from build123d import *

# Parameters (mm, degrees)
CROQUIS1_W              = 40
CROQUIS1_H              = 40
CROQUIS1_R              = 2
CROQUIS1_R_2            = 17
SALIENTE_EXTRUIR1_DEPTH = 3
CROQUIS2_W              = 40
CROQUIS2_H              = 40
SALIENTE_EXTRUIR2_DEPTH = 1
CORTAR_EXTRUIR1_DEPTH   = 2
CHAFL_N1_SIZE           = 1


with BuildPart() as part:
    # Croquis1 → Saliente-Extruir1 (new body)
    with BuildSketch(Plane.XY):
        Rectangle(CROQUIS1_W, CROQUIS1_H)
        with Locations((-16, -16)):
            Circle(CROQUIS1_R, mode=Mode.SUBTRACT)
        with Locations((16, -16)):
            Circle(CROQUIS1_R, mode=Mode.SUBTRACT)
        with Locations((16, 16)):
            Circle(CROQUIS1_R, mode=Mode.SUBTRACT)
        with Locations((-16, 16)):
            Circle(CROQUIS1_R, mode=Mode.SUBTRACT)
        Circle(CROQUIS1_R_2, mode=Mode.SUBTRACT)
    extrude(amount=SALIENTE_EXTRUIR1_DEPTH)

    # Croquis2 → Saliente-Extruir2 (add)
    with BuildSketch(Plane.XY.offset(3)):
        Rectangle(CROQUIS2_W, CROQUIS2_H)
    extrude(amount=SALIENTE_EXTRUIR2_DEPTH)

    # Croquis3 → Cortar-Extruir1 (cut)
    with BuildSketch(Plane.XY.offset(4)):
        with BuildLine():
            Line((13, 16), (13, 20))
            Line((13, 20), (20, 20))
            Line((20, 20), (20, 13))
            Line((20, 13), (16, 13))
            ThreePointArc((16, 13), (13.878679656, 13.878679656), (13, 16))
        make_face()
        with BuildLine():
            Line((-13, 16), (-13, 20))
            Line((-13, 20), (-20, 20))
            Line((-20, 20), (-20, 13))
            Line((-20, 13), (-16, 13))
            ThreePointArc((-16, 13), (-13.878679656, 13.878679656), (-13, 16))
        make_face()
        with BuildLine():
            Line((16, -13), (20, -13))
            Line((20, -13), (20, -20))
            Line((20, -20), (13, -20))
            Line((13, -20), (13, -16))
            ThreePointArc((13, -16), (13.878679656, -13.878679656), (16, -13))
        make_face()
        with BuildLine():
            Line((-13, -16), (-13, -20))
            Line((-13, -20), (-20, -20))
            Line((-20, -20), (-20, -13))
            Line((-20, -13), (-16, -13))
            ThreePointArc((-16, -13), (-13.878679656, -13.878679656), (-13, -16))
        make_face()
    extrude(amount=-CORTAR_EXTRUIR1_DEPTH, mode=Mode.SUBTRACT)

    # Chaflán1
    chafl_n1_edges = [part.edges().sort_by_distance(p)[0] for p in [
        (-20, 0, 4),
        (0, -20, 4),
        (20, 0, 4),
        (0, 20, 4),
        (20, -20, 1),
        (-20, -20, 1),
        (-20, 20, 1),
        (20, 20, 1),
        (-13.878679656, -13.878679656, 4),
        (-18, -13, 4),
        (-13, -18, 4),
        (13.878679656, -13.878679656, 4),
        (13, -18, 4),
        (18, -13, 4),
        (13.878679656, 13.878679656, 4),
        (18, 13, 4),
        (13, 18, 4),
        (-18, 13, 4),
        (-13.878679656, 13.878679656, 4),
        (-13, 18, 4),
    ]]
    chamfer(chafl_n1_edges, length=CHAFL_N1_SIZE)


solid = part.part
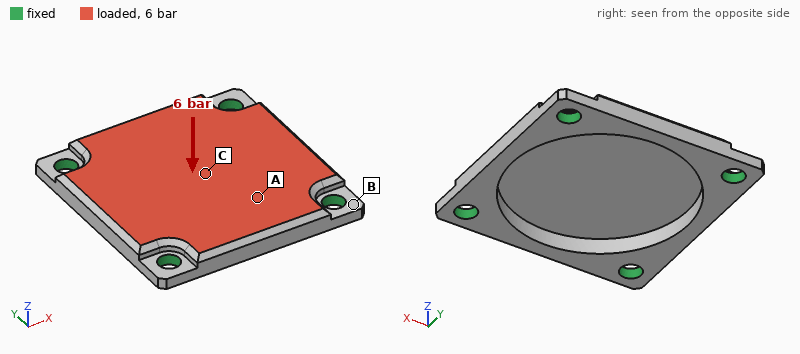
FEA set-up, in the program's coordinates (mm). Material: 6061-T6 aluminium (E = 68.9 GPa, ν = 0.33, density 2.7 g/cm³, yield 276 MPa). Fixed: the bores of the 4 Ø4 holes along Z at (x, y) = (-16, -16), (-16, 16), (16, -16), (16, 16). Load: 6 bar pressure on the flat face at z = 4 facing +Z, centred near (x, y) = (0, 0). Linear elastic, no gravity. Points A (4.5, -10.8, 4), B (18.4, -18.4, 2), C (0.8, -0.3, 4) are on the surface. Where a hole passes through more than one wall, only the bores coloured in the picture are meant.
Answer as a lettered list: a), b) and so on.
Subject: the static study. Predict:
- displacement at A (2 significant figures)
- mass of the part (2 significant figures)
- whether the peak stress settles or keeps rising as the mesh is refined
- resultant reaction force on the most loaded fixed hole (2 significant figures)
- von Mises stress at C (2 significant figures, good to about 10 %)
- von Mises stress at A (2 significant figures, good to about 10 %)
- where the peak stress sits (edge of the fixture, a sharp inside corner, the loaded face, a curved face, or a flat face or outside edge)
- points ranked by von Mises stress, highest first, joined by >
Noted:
a) 0.058 mm
b) 8.4 g
c) keeps rising
d) 340 N
e) 100 MPa
f) 44 MPa
g) edge of the fixture
h) C > A > B
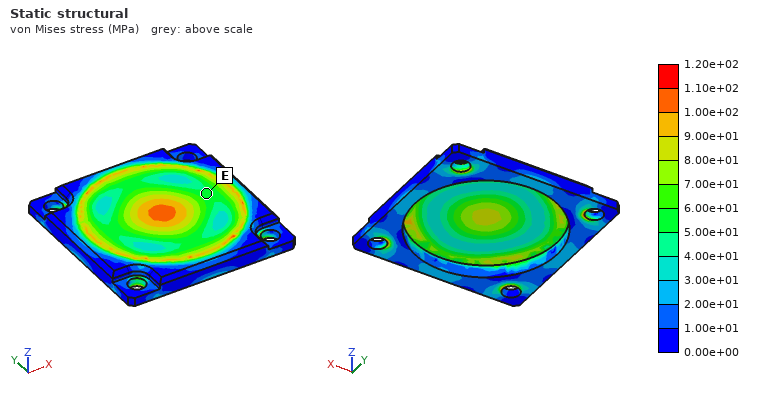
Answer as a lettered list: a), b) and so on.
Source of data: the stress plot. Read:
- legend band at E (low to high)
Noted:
a) 5.00e+01 to 6.00e+01 MPa
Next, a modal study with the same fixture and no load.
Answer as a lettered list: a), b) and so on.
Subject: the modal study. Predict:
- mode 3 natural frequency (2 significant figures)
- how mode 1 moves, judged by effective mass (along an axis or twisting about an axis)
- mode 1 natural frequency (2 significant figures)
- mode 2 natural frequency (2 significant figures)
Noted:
a) 15 kHz
b) along Z
c) 7700 Hz
d) 15 kHz
